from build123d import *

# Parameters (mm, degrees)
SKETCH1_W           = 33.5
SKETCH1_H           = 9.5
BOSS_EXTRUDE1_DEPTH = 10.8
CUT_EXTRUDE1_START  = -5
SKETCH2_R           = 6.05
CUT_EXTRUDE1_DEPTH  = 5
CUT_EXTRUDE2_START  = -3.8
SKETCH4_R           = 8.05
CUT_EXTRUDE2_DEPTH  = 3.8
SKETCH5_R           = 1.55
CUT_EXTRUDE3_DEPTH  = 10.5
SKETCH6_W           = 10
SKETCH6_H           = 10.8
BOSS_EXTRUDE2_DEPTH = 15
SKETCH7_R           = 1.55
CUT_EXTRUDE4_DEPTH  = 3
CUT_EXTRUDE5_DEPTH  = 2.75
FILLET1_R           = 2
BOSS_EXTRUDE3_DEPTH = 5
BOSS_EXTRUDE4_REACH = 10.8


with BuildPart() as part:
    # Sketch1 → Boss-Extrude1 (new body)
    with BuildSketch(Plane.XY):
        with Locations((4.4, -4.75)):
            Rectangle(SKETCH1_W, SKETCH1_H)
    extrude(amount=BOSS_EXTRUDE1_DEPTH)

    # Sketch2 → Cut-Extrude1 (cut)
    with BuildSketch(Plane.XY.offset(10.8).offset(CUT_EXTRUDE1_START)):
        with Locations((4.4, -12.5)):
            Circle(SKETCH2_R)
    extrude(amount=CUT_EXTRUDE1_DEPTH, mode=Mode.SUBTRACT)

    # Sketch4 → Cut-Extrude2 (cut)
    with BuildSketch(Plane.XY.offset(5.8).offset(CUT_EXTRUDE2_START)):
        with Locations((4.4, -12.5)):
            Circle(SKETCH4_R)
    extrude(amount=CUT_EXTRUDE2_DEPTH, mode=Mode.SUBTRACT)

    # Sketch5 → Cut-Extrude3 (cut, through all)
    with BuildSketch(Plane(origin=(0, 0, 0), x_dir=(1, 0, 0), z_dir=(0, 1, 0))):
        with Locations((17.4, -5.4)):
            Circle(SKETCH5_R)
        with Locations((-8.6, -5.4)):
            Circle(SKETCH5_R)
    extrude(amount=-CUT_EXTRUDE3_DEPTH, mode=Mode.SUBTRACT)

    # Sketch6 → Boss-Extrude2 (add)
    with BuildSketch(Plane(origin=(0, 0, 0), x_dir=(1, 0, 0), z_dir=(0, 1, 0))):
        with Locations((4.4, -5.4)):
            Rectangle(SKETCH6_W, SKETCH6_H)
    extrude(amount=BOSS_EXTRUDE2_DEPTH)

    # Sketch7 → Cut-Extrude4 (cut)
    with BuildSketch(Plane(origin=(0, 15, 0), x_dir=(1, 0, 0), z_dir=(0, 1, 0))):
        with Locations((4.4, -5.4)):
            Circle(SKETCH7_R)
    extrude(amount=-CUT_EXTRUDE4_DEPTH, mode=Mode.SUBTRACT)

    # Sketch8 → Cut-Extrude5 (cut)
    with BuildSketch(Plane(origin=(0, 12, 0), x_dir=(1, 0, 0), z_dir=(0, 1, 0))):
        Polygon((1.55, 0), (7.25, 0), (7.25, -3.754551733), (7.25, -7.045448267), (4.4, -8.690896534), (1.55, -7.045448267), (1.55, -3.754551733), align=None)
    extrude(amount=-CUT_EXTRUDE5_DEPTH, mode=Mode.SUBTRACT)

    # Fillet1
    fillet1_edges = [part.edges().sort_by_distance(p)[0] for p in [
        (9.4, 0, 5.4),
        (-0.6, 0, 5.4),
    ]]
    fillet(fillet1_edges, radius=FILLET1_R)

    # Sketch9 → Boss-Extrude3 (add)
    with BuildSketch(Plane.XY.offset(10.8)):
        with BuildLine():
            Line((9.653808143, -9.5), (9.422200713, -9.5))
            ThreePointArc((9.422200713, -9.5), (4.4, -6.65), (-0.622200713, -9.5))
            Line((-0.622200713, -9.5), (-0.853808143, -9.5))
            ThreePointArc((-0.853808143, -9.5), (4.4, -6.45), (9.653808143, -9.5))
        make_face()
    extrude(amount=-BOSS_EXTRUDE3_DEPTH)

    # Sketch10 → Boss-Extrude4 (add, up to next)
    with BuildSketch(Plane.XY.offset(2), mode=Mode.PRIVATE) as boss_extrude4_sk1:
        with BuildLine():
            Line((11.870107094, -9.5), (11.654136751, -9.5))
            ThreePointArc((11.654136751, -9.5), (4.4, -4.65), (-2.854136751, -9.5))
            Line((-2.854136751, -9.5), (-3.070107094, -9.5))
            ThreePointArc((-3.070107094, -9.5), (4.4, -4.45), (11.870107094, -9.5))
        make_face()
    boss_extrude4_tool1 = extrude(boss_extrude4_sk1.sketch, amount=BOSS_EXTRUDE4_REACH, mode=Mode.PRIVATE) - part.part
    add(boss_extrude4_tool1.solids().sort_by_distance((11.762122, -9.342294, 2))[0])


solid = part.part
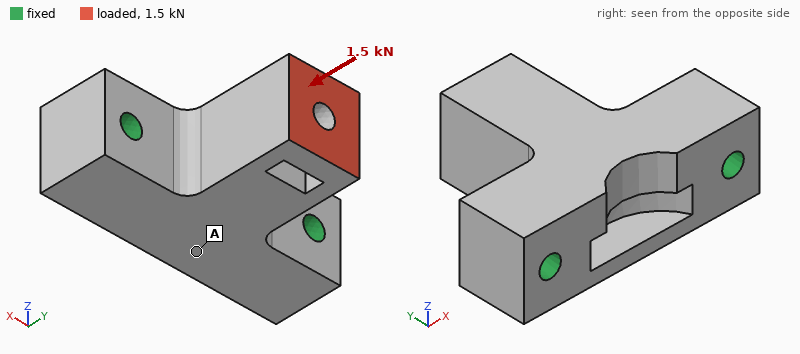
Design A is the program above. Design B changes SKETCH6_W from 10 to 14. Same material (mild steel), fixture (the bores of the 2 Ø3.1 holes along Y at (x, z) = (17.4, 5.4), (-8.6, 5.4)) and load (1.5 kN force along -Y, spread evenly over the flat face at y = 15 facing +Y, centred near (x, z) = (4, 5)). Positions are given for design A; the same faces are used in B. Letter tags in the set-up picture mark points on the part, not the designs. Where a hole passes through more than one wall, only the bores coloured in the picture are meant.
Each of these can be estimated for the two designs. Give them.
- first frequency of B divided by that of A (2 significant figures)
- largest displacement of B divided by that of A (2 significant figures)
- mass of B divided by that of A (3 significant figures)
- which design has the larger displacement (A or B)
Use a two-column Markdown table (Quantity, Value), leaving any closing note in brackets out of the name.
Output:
| Quantity | Value |
|---|---|
| first frequency of B divided by that of A | 0.94 |
| largest displacement of B divided by that of A | 0.64 |
| mass of B divided by that of A | 1.14 |
| which design has the larger displacement | A |
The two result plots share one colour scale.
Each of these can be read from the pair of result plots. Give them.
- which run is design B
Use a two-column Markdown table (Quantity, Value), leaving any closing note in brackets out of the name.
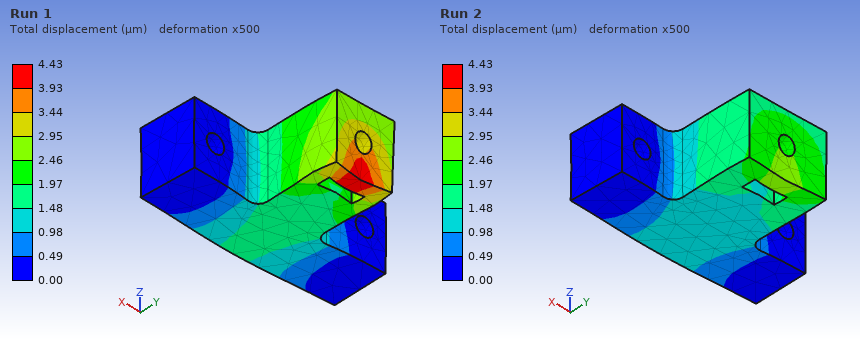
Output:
| Quantity | Value |
|---|---|
| which run is design B | Run 2 |
